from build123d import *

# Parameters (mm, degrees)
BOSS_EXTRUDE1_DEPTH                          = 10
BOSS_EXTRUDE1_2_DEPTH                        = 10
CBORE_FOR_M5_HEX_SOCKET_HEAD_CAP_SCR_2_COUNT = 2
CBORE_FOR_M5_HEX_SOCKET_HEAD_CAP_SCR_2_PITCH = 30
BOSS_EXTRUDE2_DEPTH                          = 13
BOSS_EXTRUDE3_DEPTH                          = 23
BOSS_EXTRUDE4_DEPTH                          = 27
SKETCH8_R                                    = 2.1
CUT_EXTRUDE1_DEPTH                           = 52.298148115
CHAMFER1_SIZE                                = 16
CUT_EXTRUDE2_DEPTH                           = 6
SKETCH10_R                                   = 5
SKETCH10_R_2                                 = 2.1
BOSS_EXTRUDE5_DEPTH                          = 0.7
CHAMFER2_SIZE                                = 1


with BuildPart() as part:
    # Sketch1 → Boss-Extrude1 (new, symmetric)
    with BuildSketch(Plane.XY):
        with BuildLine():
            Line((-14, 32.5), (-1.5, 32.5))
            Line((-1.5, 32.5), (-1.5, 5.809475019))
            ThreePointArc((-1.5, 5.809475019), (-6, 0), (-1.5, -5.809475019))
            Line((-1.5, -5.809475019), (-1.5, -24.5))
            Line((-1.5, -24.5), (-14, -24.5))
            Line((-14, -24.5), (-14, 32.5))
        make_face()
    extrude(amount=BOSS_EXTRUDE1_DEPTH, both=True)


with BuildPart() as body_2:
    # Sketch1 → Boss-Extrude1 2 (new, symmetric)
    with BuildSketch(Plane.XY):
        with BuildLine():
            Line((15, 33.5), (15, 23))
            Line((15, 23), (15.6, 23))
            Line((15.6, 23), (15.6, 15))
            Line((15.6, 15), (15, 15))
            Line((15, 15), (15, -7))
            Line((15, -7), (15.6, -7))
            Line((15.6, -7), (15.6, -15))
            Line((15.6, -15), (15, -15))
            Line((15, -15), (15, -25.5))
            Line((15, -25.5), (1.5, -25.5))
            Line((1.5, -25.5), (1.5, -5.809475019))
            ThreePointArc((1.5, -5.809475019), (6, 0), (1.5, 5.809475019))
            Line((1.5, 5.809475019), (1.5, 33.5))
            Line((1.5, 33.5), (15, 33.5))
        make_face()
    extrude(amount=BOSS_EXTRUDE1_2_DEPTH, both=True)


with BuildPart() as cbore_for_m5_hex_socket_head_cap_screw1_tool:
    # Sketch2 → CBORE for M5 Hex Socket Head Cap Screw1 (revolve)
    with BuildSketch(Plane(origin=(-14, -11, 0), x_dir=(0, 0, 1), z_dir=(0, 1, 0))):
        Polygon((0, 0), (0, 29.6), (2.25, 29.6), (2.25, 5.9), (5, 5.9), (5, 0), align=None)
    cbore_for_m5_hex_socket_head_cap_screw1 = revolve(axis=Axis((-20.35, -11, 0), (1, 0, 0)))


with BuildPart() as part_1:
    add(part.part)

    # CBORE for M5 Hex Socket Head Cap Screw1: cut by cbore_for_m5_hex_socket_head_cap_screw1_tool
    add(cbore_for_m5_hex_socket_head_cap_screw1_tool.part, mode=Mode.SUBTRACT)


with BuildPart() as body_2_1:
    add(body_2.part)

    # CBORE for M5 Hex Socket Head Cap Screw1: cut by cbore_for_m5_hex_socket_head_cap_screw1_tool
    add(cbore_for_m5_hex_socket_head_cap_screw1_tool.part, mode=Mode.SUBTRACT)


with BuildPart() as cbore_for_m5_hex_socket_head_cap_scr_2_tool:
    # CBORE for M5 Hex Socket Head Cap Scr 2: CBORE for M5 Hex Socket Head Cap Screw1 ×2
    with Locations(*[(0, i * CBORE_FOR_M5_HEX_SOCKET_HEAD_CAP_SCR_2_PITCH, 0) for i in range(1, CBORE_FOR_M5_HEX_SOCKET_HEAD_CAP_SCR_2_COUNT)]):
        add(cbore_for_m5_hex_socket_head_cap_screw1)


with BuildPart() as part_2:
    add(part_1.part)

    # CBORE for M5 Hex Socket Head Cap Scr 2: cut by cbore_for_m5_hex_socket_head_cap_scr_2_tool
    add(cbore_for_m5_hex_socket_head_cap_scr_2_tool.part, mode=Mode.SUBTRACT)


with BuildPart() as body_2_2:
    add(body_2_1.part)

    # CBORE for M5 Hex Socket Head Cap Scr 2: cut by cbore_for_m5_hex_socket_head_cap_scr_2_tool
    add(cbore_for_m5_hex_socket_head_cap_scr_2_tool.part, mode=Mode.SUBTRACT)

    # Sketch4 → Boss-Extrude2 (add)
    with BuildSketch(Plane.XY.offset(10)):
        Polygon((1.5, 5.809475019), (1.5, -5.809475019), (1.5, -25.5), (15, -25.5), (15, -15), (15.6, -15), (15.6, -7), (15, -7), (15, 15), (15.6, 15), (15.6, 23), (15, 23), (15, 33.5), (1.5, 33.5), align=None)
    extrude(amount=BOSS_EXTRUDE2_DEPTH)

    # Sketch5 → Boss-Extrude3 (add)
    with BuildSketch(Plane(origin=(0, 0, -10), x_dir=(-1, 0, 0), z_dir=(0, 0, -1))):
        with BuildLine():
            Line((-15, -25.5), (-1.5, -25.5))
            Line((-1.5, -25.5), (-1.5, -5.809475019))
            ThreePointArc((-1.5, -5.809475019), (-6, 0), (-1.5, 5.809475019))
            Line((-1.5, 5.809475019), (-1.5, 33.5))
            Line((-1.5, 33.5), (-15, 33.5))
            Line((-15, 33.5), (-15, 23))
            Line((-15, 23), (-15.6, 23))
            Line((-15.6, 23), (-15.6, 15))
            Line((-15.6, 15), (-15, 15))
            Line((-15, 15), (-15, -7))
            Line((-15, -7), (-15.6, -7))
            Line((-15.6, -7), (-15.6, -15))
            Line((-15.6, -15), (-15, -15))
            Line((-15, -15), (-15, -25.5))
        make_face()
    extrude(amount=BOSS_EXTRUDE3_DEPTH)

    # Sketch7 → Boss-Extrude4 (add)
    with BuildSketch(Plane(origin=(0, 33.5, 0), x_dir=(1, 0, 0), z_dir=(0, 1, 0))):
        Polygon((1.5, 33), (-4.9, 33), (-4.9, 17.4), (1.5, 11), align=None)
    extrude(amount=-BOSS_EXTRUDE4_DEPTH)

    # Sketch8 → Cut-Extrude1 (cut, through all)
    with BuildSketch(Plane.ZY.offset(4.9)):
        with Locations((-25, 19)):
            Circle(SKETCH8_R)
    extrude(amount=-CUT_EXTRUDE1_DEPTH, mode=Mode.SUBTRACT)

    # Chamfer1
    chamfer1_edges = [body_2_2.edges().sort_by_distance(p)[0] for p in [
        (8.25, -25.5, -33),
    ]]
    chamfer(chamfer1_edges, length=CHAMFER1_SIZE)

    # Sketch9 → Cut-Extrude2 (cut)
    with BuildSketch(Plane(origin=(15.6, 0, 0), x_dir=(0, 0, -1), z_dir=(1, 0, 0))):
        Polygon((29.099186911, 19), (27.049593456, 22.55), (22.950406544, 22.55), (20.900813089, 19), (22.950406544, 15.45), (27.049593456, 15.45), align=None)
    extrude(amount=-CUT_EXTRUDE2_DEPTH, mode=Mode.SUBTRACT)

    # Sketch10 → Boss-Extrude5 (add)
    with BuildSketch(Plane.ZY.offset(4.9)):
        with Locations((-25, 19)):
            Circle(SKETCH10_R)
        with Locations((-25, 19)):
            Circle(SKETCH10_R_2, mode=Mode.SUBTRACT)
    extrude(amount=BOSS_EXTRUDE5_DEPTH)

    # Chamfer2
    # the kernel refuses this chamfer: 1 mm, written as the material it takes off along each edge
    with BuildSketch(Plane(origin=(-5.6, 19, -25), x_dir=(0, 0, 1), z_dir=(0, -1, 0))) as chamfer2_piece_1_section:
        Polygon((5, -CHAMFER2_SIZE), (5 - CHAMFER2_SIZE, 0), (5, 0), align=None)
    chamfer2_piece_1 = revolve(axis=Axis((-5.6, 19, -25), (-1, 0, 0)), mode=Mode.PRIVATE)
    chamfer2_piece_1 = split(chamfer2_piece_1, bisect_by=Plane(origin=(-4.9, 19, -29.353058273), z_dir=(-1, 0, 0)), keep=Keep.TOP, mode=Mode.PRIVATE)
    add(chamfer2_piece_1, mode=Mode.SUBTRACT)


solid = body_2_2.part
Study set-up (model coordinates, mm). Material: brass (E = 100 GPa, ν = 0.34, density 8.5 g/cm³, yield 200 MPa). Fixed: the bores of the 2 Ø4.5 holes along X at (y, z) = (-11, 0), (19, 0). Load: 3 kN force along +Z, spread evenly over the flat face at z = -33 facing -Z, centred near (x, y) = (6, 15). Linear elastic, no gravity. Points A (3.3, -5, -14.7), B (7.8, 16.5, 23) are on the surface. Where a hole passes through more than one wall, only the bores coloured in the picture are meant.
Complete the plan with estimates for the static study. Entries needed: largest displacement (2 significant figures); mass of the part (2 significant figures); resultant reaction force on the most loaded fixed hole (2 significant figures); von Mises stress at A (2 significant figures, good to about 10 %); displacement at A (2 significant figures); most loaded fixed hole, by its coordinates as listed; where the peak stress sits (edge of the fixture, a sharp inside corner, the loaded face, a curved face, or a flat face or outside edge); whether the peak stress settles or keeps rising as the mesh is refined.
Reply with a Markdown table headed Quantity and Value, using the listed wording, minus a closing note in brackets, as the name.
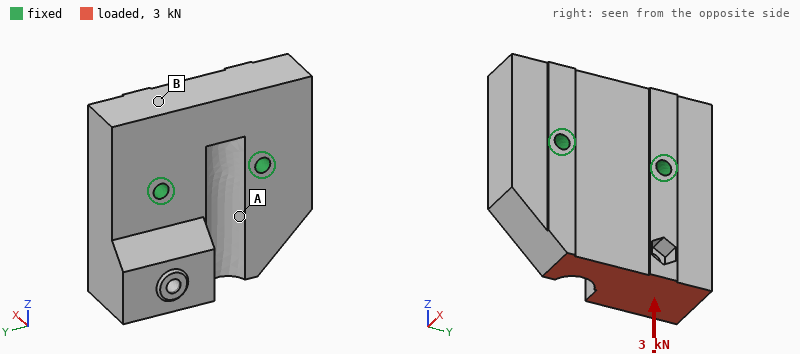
| Quantity | Value |
|---|---|
| largest displacement | 6.8 µm |
| mass of the part | 370 g |
| resultant reaction force on the most loaded fixed hole | 2.5 kN |
| von Mises stress at A | 5.0 MPa |
| displacement at A | 1.1 µm |
| most loaded fixed hole, by its coordinates as listed | (19, 0) |
| where the peak stress sits | edge of the fixture |
| whether the peak stress settles or keeps rising as the mesh is refined | keeps rising |
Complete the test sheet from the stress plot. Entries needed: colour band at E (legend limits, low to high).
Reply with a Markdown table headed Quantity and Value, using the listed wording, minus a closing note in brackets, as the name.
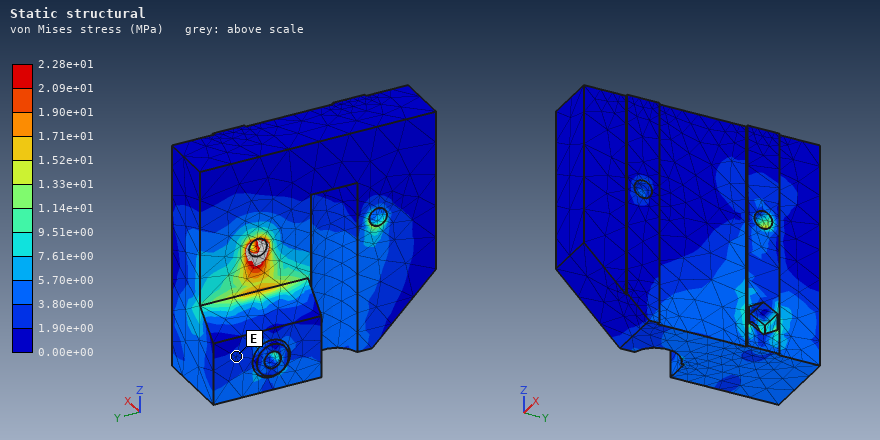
| Quantity | Value |
|---|---|
| colour band at E | 1.90e+00 to 3.80e+00 MPa |
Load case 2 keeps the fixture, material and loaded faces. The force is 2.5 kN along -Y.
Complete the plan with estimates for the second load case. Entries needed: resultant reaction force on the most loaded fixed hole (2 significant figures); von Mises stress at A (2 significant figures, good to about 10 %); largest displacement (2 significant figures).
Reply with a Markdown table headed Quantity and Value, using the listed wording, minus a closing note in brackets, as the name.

| Quantity | Value |
|---|---|
| resultant reaction force on the most loaded fixed hole | 2.8 kN |
| von Mises stress at A | 8.9 MPa |
| largest displacement | 11 µm |
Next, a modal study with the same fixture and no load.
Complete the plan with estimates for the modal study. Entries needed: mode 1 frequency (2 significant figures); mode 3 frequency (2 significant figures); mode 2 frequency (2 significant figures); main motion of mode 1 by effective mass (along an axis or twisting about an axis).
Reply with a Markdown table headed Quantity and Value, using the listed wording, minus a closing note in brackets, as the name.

| Quantity | Value |
|---|---|
| mode 1 frequency | 4900 Hz |
| mode 3 frequency | 9700 Hz |
| mode 2 frequency | 8300 Hz |
| main motion of mode 1 by effective mass | along X |
